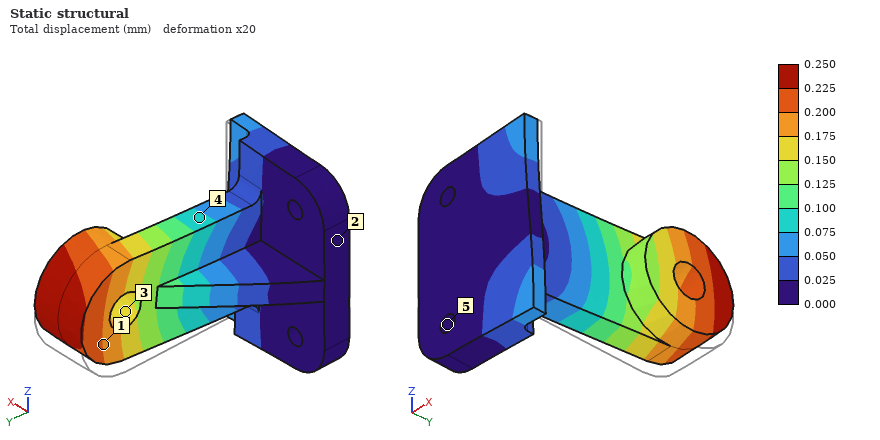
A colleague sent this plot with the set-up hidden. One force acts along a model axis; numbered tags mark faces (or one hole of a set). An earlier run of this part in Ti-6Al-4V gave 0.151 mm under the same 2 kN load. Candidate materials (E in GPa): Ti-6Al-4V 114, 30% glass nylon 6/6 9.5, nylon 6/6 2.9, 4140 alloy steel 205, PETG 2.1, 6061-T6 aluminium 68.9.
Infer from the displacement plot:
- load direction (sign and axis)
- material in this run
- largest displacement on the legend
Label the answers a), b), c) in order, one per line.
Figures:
a) +Z
b) 6061-T6 aluminium
c) 0.250 mm
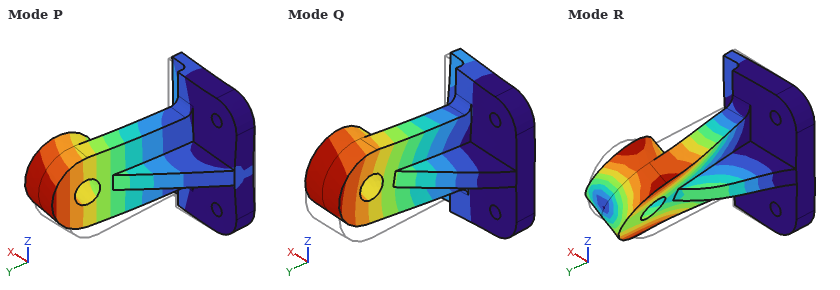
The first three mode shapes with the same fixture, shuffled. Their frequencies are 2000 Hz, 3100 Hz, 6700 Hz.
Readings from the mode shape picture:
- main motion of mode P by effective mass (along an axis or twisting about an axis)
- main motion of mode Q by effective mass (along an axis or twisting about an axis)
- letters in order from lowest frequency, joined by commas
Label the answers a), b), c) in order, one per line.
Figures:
a) along X
b) along Z
c) P, Q, R
